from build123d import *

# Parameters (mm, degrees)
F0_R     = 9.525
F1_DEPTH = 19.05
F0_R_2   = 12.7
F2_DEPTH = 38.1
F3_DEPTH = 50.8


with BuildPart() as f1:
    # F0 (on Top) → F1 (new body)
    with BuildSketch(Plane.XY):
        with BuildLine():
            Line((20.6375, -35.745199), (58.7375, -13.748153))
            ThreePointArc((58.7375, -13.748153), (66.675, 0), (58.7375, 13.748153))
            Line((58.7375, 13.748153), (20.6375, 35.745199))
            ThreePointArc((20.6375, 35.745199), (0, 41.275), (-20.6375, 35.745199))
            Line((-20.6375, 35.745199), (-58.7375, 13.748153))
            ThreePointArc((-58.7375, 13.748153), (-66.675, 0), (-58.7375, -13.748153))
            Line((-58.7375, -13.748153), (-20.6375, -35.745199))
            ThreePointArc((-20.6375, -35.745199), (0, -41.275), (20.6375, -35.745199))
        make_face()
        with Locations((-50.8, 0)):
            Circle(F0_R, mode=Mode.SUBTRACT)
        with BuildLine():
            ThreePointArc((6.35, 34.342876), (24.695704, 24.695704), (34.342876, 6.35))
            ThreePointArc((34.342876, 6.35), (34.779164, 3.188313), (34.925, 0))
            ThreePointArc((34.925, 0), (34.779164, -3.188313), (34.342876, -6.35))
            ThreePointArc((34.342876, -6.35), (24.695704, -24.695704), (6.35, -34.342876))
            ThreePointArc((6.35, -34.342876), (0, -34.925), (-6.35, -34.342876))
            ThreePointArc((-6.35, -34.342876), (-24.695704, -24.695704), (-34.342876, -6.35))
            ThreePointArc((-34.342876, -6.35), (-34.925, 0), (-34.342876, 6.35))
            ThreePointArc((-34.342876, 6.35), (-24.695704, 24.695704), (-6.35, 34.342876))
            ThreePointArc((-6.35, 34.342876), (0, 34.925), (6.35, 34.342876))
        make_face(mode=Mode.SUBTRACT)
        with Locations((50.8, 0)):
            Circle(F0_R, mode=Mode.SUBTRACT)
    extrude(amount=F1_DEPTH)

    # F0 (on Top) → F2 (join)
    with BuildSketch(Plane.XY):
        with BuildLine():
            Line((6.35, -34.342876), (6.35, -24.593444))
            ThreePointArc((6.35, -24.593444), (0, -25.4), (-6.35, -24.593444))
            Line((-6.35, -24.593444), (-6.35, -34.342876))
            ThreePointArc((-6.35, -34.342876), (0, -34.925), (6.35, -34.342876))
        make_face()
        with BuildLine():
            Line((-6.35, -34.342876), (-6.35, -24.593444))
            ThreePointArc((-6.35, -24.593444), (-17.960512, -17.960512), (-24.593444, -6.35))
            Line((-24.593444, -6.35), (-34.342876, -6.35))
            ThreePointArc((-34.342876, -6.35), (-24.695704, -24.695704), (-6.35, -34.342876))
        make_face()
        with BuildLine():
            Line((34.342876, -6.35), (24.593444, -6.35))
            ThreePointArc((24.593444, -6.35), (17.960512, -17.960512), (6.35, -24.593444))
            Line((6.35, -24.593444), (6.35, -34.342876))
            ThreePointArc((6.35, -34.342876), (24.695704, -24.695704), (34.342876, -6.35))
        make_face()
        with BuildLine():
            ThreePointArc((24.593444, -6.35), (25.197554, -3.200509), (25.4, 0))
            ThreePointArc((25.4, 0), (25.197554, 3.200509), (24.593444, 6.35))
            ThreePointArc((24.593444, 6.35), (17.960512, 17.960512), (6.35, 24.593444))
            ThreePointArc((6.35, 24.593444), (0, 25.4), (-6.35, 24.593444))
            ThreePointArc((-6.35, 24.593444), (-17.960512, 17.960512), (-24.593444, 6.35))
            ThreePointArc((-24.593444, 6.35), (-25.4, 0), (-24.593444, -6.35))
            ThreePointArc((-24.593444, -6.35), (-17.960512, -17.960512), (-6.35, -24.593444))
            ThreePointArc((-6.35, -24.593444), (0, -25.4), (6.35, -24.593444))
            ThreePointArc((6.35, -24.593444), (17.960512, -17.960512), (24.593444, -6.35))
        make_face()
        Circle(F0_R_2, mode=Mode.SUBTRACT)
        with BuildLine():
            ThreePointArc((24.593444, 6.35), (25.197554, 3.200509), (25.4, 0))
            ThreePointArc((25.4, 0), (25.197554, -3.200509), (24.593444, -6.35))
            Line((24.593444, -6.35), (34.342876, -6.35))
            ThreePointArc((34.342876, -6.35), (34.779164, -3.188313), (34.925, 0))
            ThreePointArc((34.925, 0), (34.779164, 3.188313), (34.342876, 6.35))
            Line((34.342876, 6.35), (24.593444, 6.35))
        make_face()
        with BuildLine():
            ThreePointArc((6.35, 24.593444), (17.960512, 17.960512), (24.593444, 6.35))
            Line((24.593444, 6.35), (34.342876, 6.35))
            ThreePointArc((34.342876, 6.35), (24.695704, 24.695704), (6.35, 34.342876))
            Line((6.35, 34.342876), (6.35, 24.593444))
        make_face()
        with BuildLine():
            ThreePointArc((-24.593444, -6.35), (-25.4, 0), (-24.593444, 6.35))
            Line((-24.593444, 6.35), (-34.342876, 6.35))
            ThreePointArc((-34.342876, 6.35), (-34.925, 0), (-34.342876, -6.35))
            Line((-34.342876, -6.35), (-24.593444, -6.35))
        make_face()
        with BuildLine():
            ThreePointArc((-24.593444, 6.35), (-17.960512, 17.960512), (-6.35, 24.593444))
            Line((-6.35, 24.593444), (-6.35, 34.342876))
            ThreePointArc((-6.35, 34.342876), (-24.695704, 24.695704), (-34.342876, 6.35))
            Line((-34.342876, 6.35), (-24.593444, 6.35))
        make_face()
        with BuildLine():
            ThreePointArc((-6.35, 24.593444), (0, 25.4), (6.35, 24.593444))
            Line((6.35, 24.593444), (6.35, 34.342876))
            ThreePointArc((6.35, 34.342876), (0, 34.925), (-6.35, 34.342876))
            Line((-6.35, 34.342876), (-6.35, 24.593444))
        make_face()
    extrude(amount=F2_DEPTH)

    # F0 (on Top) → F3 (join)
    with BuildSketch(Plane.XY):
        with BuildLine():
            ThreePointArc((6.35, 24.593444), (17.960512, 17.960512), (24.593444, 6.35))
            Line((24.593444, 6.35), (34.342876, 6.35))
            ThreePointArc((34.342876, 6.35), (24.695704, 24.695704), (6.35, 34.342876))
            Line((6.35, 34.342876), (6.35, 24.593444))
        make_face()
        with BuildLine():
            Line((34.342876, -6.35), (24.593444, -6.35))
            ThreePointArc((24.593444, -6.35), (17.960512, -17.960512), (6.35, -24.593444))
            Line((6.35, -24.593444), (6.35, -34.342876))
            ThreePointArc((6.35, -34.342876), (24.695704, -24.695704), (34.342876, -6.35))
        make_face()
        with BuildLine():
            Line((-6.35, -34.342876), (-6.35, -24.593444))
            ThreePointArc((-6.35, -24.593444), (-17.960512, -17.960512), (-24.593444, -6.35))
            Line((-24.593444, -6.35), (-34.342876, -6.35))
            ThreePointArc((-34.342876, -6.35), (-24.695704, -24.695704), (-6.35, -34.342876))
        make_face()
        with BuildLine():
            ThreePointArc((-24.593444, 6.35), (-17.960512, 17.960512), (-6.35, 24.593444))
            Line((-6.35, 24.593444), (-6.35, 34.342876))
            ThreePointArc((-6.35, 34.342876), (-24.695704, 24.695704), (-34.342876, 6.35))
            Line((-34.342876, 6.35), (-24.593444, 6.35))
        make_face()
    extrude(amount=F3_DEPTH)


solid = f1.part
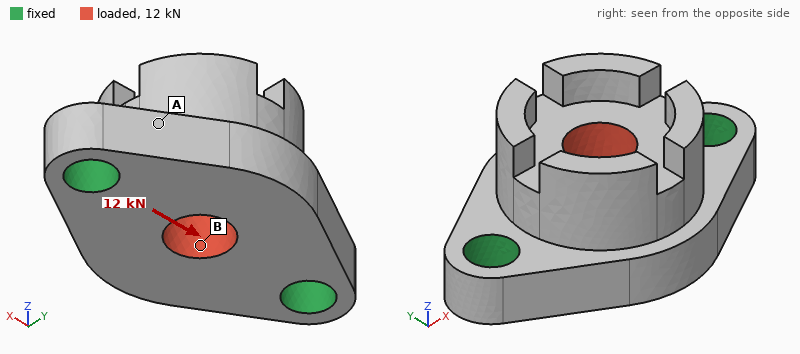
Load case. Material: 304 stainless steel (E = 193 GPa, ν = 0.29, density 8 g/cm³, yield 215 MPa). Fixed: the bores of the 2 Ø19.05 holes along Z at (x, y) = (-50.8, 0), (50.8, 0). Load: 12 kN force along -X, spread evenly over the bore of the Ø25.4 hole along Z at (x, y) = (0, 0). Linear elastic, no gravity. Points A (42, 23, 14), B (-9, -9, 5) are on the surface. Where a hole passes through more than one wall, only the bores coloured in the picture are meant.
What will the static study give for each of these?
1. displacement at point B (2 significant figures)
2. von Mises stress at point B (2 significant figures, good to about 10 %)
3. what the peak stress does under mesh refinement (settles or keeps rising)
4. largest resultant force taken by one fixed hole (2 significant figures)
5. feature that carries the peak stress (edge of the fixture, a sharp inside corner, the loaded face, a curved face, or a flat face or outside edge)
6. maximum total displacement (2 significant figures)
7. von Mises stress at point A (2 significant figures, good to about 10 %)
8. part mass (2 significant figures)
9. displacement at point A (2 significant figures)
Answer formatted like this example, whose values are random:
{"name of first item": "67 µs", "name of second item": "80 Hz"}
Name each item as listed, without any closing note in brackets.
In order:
{"displacement at point B": "1.2 µm", "von Mises stress at point B": "6.2 MPa", "what the peak stress does under mesh refinement": "keeps rising", "largest resultant force taken by one fixed hole": "6.1 kN", "feature that carries the peak stress": "a sharp inside corner", "maximum total displacement": "2.0 µm", "von Mises stress at point A": "2.9 MPa", "part mass": "1.6 kg", "displacement at point A": "0.76 µm"}
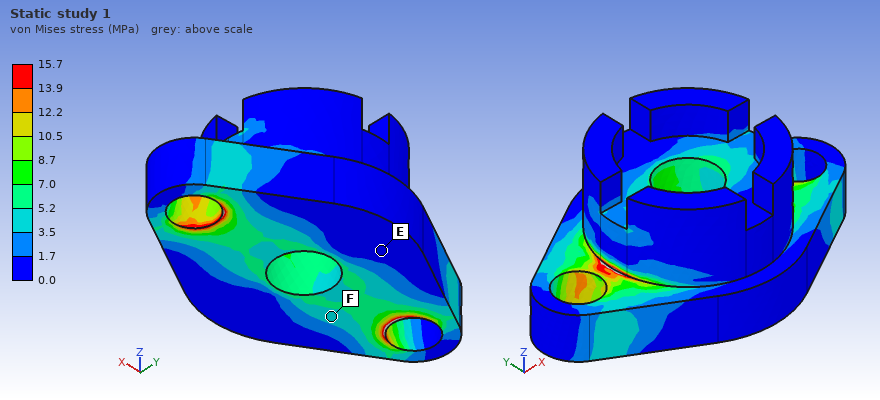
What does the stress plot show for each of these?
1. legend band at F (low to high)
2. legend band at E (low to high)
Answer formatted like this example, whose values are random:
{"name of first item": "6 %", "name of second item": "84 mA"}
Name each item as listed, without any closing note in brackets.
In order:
{"legend band at F": "3.5 to 5.2 MPa", "legend band at E": "0.0 to 1.7 MPa"}
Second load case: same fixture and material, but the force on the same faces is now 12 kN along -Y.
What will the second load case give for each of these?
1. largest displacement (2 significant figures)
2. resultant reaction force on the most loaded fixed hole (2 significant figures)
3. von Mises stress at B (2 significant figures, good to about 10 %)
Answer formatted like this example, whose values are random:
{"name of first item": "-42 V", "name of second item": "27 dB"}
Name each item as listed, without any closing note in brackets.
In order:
{"largest displacement": "10.0 µm", "resultant reaction force on the most loaded fixed hole": "6.0 kN", "von Mises stress at B": "5.8 MPa"}
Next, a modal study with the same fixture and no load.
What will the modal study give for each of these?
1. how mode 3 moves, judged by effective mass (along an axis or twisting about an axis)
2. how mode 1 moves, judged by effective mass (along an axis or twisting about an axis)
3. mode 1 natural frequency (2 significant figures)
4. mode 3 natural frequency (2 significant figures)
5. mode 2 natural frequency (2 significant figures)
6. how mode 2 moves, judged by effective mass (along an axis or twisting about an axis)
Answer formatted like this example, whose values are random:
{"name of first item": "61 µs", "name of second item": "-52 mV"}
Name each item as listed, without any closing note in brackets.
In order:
{"how mode 3 moves, judged by effective mass": "along Y", "how mode 1 moves, judged by effective mass": "along Y", "mode 1 natural frequency": "4500 Hz", "mode 3 natural frequency": "11 kHz", "mode 2 natural frequency": "7200 Hz", "how mode 2 moves, judged by effective mass": "along Z"}
